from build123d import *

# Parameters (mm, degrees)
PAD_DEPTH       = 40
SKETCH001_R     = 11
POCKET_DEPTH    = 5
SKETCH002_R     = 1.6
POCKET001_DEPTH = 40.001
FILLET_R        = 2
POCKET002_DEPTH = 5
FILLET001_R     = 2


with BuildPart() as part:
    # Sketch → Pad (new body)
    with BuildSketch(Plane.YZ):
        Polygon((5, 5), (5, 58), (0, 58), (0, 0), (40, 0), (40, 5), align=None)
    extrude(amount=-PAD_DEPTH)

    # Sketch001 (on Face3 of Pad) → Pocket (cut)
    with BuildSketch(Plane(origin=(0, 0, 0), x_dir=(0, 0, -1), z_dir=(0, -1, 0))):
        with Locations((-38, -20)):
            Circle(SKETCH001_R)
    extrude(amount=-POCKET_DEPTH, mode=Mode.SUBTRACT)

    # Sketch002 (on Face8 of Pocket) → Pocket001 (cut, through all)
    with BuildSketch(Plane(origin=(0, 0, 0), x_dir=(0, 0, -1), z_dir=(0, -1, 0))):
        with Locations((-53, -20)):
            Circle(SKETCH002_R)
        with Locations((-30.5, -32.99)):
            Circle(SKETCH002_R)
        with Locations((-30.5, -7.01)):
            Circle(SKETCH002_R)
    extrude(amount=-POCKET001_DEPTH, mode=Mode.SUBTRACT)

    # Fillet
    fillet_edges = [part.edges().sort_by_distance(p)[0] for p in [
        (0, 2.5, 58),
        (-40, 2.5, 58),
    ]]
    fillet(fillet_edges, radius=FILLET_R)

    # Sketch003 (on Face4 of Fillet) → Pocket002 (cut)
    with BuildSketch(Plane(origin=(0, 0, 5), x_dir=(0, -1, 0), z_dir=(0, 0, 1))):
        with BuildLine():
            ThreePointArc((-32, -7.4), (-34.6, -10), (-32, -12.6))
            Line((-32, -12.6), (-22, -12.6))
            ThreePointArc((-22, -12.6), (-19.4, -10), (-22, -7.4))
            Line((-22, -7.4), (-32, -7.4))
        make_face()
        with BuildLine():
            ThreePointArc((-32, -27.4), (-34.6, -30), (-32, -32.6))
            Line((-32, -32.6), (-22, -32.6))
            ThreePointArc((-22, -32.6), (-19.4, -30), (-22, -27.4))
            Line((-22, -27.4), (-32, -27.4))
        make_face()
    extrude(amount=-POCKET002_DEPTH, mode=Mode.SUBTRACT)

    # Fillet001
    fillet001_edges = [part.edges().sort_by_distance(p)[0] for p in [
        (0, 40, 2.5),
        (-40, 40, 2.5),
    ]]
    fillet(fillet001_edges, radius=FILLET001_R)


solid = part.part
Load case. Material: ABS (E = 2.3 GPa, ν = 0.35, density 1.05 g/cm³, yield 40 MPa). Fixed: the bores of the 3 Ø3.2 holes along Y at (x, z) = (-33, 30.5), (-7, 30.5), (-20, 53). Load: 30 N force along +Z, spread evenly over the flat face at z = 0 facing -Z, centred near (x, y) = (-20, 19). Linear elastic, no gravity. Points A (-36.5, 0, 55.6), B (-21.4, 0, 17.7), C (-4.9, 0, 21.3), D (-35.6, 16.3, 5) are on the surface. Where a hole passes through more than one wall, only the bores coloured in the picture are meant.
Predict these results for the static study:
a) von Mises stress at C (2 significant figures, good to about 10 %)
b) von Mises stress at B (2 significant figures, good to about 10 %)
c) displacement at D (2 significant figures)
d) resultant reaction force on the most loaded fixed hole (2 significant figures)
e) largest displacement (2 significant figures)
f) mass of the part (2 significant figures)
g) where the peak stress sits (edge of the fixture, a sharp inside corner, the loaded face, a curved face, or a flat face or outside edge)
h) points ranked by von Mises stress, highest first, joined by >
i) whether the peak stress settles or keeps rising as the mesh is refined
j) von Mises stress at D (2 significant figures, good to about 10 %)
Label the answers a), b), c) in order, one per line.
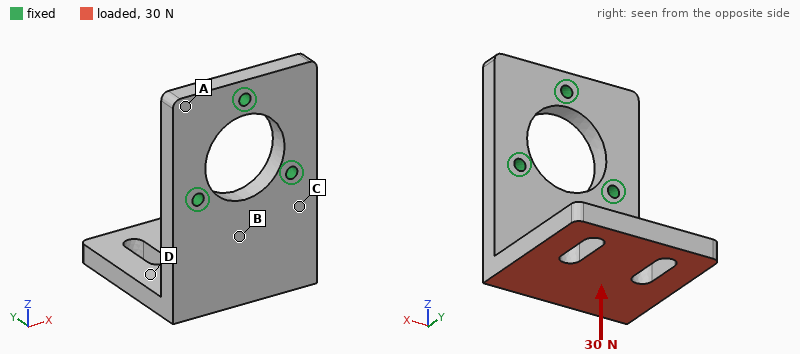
a) 3.2 MPa
b) 2.1 MPa
c) 0.32 mm
d) 16 N
e) 0.81 mm
f) 17 g
g) edge of the fixture
h) C > B > D > A
i) keeps rising
j) 1.2 MPa
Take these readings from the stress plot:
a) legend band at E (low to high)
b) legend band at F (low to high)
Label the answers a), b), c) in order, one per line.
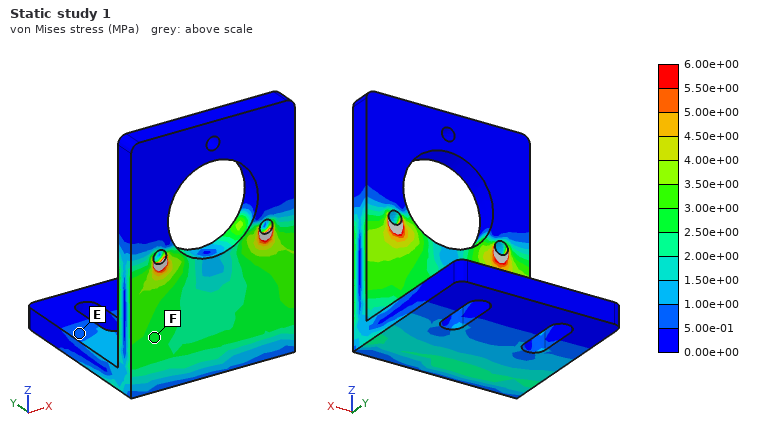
a) 5.00e-01 to 1.00e+00 MPa
b) 2.50e+00 to 3.00e+00 MPa
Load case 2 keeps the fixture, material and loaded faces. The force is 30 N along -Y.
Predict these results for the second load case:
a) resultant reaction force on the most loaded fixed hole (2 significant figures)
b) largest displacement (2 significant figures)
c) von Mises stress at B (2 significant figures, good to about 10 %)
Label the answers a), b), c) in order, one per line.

a) 16 N
b) 0.79 mm
c) 2.2 MPa
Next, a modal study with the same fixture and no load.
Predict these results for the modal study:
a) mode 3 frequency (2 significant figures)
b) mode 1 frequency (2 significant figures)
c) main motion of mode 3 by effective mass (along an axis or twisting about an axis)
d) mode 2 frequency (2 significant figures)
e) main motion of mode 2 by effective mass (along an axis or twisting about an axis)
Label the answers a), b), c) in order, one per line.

a) 1000 Hz
b) 360 Hz
c) along Y
d) 690 Hz
e) along X
